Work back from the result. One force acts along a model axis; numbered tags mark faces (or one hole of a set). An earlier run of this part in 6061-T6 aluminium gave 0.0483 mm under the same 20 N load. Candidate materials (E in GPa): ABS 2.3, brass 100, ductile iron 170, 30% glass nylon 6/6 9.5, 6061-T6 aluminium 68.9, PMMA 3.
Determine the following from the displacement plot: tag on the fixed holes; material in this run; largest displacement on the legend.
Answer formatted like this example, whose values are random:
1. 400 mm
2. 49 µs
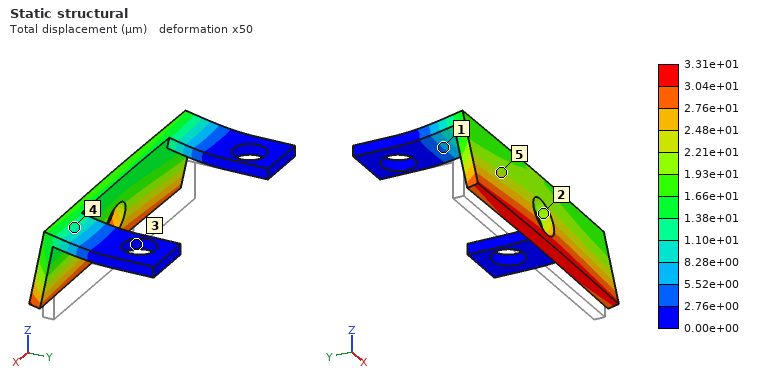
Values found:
1. 3
2. brass
3. 3.31e+01 µm
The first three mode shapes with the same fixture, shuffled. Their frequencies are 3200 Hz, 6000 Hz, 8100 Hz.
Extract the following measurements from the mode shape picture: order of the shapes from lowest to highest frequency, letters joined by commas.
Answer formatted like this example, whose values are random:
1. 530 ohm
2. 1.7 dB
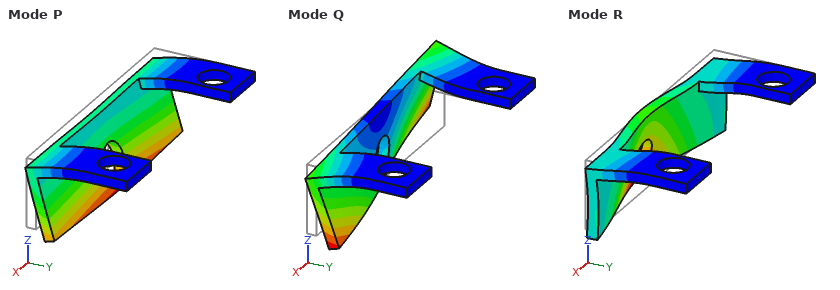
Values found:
1. P, Q, R
